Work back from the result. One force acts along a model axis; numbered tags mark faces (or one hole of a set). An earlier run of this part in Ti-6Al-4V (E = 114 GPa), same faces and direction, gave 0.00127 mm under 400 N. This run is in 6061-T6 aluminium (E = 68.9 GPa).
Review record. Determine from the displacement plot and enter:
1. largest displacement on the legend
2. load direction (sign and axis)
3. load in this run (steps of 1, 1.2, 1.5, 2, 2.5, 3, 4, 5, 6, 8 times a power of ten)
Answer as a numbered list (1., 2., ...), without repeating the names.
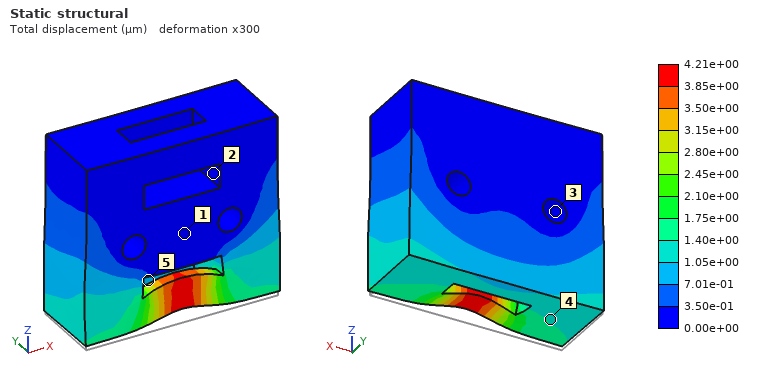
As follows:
1. 4.21e+00 µm
2. +Z
3. 800 N
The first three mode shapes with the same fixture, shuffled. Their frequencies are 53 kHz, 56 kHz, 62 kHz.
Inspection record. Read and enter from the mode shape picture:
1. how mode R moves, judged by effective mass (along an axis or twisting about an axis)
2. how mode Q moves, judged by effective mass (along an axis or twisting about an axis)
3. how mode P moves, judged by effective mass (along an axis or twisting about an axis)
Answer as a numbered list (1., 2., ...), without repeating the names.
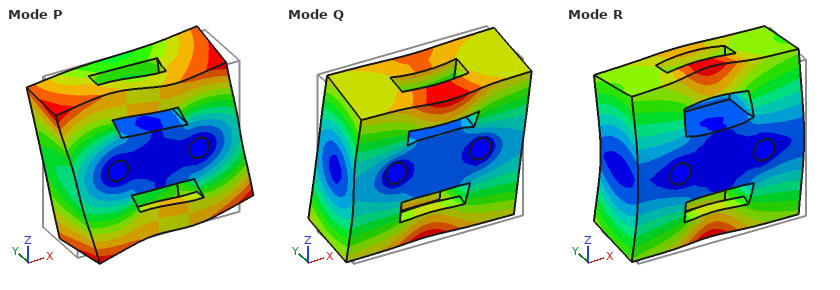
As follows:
1. along Y
2. twisting about X
3. twisting about Y
